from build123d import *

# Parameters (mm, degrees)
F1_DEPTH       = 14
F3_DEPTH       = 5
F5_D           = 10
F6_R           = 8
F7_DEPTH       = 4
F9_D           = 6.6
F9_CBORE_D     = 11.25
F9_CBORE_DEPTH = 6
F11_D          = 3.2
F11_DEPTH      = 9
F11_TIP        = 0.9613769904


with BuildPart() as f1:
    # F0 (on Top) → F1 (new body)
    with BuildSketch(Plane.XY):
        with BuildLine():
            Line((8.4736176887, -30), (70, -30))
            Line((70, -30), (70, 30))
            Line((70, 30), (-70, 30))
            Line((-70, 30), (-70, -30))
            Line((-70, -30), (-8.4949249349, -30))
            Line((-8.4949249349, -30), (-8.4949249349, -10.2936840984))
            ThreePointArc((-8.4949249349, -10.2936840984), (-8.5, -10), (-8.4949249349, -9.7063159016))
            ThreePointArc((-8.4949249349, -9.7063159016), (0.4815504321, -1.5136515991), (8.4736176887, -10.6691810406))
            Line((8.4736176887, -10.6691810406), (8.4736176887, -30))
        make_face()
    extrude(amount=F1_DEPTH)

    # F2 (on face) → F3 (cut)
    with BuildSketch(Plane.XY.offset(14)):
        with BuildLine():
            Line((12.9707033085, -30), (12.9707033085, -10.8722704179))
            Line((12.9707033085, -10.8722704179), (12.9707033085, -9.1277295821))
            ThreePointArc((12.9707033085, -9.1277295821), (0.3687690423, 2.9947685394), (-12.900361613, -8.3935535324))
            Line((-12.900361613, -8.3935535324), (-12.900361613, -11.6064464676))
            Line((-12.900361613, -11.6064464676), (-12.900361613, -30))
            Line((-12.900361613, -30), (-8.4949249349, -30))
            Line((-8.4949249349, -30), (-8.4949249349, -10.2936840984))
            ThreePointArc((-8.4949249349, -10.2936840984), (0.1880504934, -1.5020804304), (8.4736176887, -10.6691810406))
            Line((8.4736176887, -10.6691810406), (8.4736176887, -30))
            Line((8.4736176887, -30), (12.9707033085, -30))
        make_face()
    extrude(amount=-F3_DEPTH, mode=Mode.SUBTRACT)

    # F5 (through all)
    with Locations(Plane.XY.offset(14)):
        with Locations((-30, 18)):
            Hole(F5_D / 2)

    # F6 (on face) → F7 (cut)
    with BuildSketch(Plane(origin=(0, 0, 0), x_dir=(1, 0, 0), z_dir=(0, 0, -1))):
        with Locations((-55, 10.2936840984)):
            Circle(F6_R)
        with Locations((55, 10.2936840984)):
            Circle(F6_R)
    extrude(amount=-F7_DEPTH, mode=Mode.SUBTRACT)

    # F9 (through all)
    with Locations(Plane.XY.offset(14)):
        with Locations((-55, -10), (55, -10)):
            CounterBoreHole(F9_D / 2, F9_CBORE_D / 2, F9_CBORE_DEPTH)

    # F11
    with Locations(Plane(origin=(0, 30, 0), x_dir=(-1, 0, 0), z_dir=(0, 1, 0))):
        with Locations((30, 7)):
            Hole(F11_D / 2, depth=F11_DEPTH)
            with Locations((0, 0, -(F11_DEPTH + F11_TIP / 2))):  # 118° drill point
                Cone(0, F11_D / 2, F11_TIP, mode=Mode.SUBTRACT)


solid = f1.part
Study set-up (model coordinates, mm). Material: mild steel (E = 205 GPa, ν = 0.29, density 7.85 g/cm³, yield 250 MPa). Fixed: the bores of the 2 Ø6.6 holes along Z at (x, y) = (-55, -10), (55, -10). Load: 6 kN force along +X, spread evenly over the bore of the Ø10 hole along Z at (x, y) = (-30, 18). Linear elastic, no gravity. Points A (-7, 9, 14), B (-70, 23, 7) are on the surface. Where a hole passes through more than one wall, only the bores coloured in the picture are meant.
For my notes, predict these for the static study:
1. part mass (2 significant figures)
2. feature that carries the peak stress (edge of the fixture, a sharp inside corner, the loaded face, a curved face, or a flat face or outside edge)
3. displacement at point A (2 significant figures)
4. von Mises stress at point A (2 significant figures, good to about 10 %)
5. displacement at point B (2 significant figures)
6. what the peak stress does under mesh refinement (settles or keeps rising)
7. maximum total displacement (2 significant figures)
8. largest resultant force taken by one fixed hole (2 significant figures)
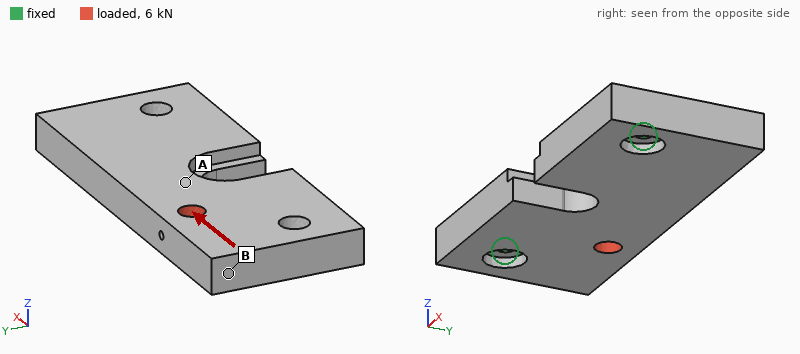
830 g
edge of the fixture
3.2 µm
11 MPa
5.1 µm
keeps rising
5.8 µm
3.4 kN
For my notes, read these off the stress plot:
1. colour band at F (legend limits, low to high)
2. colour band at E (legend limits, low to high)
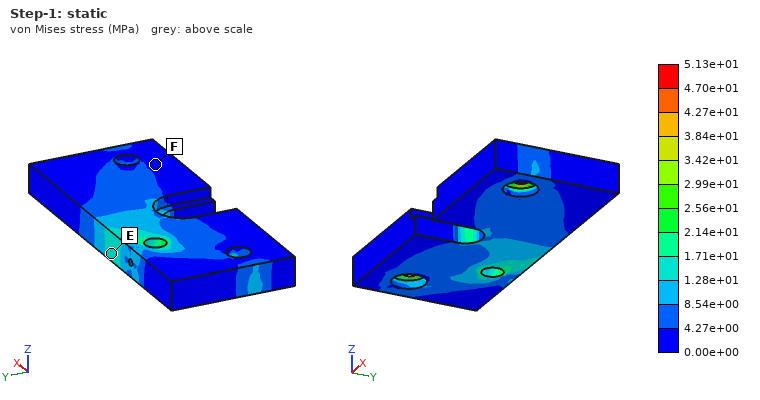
0.00e+00 to 4.27e+00 MPa
1.28e+01 to 1.71e+01 MPa
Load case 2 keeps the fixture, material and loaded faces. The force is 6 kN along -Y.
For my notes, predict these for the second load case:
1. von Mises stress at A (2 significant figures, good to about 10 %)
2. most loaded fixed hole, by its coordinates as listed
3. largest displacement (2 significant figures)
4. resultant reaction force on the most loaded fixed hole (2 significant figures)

9.7 MPa
(-55, -10)
11 µm
5.2 kN
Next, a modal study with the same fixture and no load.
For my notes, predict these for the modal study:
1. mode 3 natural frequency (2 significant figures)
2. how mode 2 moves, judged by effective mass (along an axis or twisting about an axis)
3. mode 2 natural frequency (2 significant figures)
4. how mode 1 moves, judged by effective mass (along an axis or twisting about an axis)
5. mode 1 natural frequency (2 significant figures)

3800 Hz
along Z
3000 Hz
along Z
1600 Hz
